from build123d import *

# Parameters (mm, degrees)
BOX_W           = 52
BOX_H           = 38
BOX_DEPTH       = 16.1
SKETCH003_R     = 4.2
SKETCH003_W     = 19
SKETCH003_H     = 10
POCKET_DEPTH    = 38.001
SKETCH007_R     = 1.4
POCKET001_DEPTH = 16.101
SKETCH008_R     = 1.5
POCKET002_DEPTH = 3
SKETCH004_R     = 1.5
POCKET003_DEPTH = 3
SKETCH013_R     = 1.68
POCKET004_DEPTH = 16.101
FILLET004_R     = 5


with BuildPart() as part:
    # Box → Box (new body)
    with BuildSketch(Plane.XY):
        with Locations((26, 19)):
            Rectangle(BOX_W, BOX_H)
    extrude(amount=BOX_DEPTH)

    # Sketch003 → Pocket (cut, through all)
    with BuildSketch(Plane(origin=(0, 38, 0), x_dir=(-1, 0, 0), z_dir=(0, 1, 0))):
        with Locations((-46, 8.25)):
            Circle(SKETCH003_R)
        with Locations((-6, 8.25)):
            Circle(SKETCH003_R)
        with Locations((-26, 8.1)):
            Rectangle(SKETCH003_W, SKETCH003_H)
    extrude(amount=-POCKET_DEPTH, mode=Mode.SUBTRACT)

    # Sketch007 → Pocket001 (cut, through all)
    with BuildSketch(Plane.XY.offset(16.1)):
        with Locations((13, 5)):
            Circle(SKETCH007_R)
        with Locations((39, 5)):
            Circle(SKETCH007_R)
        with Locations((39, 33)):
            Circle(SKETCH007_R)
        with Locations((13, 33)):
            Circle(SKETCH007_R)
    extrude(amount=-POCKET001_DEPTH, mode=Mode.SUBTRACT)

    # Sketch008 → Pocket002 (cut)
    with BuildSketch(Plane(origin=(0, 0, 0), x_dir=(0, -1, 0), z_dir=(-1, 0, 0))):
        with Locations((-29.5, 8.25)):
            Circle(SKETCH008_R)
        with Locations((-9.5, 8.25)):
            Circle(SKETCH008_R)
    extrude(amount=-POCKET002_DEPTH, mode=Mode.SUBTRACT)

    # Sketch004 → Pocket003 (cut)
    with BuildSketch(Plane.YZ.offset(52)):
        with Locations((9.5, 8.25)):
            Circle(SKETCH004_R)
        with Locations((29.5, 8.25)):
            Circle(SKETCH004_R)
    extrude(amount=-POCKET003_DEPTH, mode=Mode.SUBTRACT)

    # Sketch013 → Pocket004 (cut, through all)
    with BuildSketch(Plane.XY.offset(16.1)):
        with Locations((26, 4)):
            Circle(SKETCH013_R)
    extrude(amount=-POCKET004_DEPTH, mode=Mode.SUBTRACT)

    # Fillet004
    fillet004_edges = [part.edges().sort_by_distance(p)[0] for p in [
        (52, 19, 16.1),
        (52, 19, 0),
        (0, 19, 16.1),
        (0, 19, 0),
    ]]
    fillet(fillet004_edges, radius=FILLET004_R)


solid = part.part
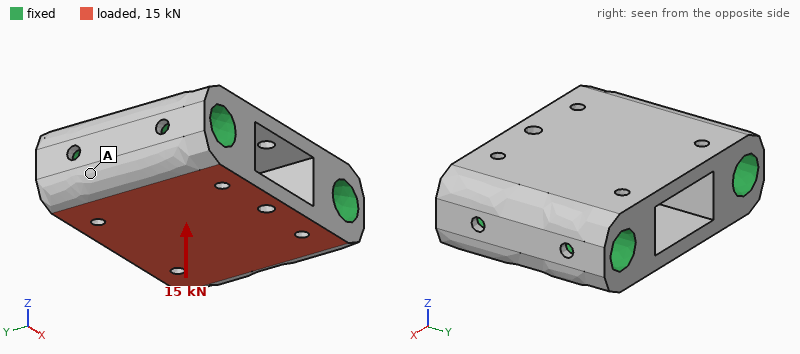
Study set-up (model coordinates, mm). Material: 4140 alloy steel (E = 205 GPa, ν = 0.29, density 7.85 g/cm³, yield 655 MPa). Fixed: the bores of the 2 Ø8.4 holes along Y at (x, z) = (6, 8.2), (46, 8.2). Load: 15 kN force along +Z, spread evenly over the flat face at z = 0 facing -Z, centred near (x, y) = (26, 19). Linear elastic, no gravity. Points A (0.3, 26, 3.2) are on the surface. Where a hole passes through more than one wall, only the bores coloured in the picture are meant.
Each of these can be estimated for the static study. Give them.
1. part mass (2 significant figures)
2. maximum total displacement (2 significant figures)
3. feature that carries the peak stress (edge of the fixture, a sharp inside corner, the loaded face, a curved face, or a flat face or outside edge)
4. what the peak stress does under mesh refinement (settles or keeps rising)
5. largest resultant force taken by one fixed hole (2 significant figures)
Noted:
150 g
18 µm
a sharp inside corner
keeps rising
7.7 kN
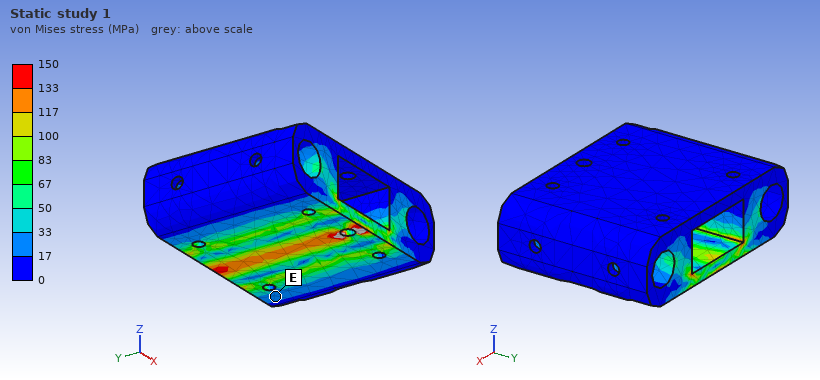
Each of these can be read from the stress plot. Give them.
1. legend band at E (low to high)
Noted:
17 to 33 MPa
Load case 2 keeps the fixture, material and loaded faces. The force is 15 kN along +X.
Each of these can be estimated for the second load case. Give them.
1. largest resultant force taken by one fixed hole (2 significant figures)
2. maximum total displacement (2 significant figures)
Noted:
7.5 kN
2.8 µm
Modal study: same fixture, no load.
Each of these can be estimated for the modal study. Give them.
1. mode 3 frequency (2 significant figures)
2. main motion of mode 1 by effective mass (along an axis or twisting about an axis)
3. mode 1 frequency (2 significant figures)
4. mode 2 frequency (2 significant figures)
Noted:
29 kHz
along Z
28 kHz
29 kHz
